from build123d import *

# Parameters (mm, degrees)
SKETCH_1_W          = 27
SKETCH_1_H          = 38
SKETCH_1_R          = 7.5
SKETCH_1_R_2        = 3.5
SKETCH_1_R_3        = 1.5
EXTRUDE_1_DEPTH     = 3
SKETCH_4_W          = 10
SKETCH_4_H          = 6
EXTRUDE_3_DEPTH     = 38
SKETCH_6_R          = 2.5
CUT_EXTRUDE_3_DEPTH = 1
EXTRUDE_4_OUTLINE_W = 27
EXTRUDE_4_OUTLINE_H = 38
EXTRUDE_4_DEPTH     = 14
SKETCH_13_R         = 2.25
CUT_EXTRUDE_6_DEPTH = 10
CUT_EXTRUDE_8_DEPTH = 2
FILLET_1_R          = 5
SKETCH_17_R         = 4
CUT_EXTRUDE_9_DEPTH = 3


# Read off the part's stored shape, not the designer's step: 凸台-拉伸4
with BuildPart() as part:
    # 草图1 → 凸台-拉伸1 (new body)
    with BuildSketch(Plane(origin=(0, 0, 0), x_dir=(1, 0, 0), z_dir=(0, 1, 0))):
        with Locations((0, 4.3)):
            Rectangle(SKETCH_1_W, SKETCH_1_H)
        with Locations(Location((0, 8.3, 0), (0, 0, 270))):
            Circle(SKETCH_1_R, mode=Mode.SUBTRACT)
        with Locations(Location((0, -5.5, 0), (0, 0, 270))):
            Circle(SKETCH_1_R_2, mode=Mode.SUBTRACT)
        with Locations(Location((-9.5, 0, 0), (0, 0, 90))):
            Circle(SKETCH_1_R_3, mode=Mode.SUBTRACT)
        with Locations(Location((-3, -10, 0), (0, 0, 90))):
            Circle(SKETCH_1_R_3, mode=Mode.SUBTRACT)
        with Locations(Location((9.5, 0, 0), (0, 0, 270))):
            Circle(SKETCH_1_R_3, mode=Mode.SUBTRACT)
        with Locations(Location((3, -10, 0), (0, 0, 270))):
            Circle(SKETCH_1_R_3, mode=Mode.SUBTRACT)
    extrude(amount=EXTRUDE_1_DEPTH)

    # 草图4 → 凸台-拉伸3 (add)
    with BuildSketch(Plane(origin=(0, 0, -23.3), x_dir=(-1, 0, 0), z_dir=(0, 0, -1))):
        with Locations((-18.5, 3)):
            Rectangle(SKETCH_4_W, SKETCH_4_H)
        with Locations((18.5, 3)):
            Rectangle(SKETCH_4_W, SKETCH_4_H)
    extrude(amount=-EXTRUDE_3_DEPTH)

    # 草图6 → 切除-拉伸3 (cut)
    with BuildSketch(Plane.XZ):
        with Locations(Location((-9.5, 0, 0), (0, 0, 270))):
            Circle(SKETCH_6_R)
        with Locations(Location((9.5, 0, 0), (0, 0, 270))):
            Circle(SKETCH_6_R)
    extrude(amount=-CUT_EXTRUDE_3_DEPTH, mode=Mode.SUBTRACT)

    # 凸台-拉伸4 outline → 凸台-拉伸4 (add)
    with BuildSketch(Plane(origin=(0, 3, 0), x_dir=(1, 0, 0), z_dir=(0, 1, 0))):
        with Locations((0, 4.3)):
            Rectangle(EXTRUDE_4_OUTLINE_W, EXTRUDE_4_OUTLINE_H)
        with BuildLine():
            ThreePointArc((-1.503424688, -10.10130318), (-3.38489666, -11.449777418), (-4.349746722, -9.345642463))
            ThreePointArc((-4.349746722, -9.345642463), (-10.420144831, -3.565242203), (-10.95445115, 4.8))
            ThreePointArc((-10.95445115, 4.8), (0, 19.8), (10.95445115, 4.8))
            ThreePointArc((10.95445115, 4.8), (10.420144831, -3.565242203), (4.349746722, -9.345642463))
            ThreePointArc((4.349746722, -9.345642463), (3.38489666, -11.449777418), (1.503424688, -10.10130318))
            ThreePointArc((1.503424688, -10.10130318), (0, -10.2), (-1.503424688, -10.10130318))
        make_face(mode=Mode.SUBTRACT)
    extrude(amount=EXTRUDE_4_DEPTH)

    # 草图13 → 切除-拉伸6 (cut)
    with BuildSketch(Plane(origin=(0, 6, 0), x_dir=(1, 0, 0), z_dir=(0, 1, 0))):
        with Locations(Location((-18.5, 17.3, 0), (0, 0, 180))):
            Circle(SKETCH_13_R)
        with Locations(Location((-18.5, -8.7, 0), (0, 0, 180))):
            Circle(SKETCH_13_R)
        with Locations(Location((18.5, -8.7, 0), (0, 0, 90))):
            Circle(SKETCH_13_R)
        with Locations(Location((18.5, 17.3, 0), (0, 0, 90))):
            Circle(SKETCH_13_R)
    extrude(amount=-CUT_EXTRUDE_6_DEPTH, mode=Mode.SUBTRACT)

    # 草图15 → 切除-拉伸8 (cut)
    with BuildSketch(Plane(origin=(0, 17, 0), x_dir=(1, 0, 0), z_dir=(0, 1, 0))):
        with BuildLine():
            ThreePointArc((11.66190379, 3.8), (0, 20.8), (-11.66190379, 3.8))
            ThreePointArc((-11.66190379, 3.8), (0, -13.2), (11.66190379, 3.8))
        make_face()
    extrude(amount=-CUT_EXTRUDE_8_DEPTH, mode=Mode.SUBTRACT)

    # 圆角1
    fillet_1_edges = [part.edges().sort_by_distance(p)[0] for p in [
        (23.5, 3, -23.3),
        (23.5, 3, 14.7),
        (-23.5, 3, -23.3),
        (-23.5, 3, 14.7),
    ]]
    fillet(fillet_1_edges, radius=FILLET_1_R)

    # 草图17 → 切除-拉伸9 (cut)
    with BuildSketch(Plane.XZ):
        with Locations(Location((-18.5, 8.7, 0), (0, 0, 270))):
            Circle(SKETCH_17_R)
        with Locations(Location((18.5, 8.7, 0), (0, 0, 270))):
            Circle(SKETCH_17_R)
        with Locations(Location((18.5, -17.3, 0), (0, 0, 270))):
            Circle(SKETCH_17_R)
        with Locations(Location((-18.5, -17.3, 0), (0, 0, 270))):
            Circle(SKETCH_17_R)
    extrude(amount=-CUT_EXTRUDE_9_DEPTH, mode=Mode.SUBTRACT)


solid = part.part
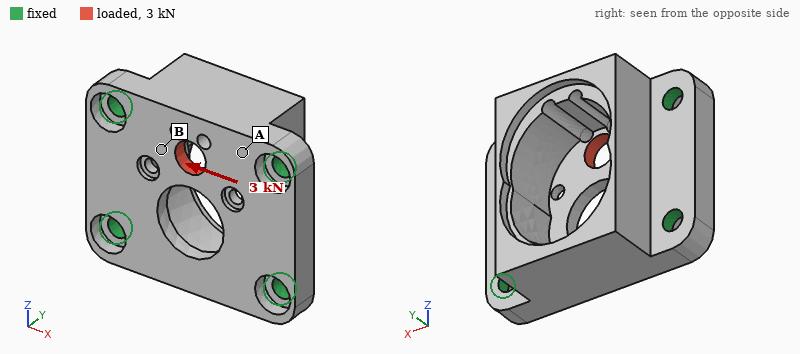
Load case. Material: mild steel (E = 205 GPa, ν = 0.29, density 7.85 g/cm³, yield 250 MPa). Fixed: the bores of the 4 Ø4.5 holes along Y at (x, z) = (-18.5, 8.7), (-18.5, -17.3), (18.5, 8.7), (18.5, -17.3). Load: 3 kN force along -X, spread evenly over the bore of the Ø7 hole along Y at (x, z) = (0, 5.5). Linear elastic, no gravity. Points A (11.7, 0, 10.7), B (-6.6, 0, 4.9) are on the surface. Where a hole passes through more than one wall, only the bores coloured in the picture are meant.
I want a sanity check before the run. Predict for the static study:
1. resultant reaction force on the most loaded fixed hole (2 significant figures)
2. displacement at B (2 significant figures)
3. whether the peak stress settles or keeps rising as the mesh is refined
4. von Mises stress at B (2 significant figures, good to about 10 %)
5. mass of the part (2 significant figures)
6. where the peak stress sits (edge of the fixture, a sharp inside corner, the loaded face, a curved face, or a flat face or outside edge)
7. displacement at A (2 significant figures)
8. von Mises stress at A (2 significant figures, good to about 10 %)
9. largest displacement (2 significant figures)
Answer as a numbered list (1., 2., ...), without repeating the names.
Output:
1. 1.3 kN
2. 2.4 µm
3. keeps rising
4. 44 MPa
5. 94 g
6. a sharp inside corner
7. 1.2 µm
8. 19 MPa
9. 4.7 µm
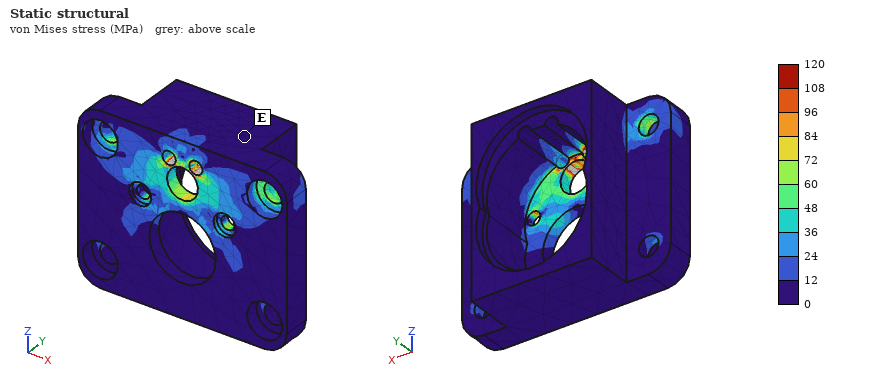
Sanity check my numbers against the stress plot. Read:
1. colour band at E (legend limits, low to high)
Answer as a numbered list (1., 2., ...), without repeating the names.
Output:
1. 0 to 12 MPa
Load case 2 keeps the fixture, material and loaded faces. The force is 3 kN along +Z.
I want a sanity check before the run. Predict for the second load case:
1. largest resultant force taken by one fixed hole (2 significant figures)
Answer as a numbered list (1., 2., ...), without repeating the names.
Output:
1. 940 N
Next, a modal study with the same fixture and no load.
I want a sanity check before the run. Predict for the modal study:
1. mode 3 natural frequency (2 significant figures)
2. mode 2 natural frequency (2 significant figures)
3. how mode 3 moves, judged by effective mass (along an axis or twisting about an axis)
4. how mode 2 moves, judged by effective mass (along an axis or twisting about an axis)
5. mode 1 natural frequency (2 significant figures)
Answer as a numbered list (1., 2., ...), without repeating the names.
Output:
1. 23 kHz
2. 17 kHz
3. along Y
4. along Y
5. 16 kHz
